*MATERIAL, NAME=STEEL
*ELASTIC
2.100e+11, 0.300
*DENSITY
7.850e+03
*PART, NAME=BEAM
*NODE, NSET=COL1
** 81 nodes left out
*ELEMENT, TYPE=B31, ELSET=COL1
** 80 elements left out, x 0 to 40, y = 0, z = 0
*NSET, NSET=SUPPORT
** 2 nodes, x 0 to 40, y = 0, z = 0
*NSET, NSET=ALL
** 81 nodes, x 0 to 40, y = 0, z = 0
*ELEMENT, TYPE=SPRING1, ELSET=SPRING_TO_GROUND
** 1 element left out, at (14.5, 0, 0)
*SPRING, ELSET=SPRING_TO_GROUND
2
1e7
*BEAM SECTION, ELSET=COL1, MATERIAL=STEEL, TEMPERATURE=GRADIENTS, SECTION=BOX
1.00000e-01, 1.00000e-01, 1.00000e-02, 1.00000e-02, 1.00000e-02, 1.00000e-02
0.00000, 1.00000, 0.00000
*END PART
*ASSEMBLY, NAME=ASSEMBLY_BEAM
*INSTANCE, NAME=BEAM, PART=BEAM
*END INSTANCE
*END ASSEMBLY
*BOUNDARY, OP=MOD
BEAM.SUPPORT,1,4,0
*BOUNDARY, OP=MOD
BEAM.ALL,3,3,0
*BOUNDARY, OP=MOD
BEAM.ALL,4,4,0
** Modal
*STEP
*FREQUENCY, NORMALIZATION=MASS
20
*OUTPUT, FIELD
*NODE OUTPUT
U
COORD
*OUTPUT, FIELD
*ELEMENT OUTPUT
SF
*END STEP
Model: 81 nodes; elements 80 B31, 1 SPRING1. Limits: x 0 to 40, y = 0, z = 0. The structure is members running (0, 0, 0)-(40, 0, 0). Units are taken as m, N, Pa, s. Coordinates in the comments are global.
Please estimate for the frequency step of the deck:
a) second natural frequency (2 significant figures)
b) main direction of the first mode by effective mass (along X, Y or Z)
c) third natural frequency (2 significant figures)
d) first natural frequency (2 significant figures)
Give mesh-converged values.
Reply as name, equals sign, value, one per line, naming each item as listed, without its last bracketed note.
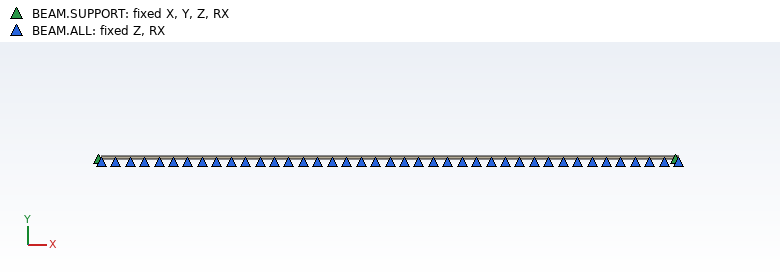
second natural frequency = 1.6 Hz
main direction of the first mode by effective mass = along Y
third natural frequency = 2.3 Hz
first natural frequency = 0.58 Hz
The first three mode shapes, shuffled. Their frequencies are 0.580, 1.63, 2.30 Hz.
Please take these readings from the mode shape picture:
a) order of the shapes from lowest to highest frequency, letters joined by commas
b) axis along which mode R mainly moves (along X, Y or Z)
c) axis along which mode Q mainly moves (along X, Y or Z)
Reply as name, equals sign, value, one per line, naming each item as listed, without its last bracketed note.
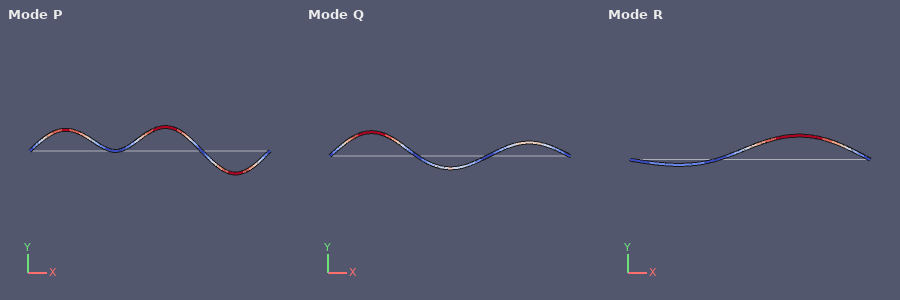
order of the shapes from lowest to highest frequency, letters joined by commas = R, Q, P
axis along which mode R mainly moves = along Y
axis along which mode Q mainly moves = along Y
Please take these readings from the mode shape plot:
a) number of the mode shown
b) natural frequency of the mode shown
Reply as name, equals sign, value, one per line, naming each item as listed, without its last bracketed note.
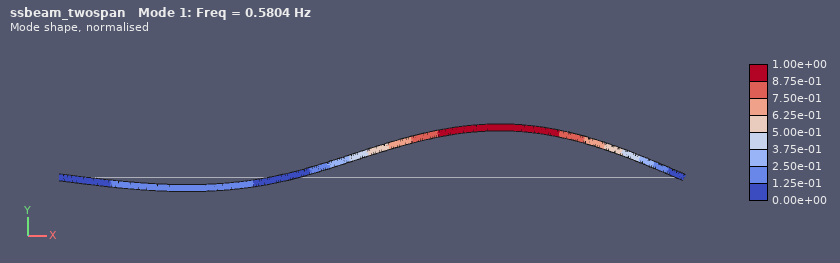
number of the mode shown = 1
natural frequency of the mode shown = 0.5804 Hz
